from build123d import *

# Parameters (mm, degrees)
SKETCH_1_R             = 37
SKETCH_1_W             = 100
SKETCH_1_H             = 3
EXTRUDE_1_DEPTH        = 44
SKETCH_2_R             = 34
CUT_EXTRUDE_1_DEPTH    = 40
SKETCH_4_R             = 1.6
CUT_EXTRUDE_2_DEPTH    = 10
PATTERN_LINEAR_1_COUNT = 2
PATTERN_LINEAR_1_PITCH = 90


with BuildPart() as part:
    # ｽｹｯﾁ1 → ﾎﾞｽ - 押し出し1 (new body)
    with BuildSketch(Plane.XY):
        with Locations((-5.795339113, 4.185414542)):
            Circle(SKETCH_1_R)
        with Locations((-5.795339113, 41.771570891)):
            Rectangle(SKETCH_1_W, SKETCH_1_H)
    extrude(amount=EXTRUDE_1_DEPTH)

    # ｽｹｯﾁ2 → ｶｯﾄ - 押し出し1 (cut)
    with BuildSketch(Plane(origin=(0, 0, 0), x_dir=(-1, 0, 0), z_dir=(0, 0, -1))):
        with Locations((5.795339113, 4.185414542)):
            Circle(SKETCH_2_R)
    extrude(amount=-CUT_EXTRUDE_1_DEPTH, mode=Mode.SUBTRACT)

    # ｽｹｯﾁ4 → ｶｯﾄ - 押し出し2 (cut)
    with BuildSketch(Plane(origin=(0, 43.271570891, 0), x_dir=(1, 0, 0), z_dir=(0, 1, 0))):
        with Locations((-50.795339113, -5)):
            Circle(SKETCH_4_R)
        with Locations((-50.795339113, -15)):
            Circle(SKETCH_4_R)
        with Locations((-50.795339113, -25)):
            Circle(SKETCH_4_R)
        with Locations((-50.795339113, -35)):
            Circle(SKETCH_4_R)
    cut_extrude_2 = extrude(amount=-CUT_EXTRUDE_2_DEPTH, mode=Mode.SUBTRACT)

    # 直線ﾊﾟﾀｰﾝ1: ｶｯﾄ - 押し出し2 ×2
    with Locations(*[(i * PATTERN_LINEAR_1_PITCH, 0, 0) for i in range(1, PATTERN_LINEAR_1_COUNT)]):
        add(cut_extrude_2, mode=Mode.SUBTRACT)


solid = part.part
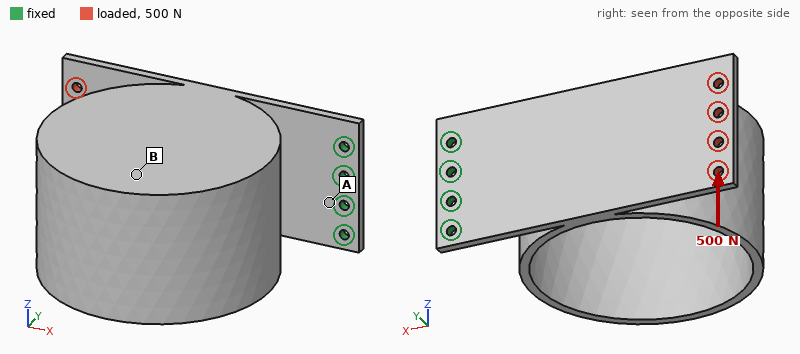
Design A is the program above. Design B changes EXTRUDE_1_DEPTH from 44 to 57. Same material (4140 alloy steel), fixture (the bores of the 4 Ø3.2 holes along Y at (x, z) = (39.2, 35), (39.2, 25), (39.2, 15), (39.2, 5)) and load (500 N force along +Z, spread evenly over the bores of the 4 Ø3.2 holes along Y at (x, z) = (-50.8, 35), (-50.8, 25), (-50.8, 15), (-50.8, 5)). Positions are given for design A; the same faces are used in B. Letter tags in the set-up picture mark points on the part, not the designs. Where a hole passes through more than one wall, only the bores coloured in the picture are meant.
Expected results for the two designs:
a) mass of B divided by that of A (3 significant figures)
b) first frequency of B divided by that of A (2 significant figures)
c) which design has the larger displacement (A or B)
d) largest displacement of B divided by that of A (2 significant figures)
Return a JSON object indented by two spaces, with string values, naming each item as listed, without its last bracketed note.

{
  "mass of B divided by that of A": "2.06",
  "first frequency of B divided by that of A": "0.77",
  "which design has the larger displacement": "A",
  "largest displacement of B divided by that of A": "0.80"
}
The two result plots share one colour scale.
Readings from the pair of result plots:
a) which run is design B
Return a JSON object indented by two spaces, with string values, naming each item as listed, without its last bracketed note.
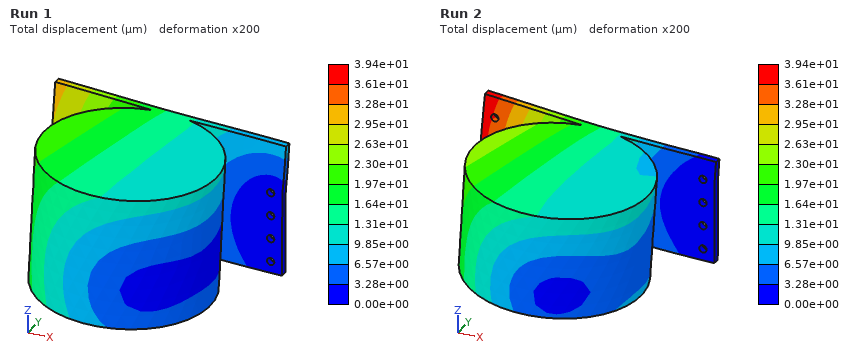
{
  "which run is design B": "Run 1"
}
